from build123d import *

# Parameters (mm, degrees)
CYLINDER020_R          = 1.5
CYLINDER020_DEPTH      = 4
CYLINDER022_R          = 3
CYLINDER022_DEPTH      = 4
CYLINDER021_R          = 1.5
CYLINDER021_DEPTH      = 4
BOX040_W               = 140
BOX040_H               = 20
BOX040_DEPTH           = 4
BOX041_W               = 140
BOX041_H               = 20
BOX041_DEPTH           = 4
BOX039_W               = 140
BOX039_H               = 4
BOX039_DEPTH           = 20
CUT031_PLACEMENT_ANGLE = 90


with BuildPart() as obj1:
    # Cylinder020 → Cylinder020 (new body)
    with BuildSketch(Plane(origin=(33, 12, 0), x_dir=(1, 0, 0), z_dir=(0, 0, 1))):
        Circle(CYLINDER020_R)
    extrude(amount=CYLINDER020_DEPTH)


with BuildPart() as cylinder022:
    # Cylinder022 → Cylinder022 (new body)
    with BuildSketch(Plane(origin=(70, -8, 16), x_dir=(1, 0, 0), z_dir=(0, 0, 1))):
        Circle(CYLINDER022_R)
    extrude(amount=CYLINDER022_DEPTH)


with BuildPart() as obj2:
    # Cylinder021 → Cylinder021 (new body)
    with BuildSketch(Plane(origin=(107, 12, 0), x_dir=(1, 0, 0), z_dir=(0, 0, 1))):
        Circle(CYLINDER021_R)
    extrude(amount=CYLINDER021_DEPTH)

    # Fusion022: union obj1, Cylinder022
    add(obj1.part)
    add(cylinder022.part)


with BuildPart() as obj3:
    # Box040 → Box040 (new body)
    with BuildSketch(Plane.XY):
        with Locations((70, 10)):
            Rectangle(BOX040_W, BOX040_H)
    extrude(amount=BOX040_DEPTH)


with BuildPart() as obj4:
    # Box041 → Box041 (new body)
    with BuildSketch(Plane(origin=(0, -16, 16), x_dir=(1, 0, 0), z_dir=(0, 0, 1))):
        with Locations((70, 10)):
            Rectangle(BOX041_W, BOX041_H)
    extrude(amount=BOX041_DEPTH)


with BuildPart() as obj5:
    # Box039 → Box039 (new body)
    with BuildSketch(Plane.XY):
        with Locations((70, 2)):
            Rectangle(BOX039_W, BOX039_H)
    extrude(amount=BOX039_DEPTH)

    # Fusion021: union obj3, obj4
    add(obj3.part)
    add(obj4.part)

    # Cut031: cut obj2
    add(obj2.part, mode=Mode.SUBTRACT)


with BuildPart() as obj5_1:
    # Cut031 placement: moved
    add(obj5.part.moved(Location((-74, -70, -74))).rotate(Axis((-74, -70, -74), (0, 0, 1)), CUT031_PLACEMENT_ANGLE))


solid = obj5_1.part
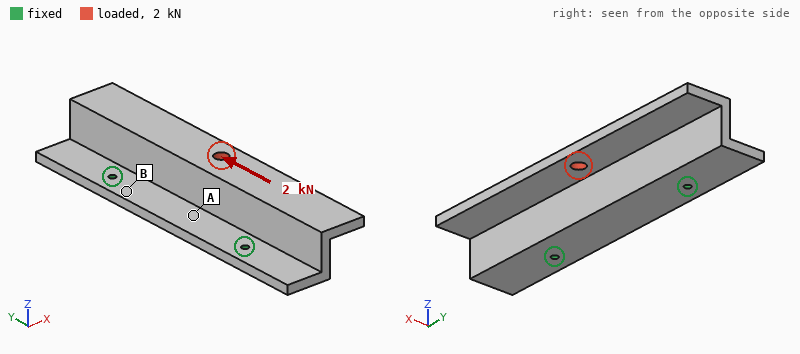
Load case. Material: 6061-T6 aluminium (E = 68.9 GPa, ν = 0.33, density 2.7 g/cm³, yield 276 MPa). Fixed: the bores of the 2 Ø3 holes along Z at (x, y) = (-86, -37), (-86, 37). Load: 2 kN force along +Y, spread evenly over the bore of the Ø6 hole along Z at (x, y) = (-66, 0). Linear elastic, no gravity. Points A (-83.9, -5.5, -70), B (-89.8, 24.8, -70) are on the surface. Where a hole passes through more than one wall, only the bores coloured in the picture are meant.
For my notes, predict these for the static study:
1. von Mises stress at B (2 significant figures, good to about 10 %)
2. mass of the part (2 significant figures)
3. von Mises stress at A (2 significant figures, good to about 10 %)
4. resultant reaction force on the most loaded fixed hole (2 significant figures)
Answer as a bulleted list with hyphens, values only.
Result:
- 14 MPa
- 78 g
- 6.9 MPa
- 1.2 kN
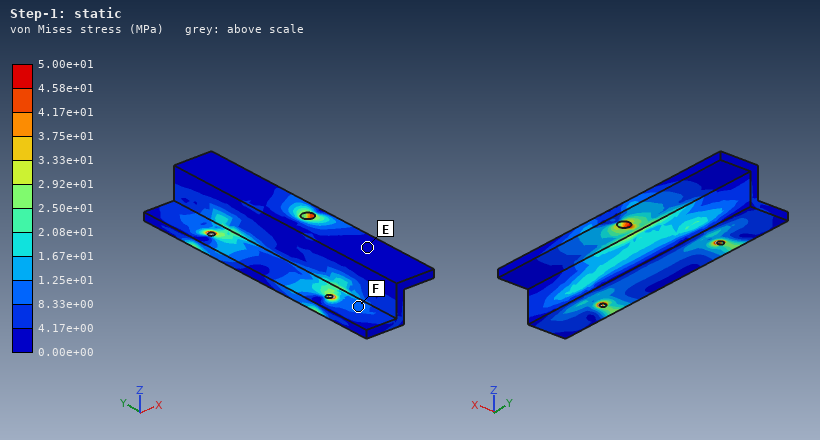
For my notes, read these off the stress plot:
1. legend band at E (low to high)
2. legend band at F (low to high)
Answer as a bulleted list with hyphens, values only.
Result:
- 0.00e+00 to 4.17e+00 MPa
- 8.33e+00 to 1.25e+01 MPa
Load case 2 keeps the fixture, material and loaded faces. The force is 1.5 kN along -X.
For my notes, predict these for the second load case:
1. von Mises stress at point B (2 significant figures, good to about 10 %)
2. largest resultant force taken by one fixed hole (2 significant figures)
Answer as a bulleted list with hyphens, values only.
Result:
- 72 MPa
- 760 N
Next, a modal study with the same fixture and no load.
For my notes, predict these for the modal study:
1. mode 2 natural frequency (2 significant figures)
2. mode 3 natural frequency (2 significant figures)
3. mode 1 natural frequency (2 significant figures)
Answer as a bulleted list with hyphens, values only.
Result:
- 2200 Hz
- 3700 Hz
- 1600 Hz
